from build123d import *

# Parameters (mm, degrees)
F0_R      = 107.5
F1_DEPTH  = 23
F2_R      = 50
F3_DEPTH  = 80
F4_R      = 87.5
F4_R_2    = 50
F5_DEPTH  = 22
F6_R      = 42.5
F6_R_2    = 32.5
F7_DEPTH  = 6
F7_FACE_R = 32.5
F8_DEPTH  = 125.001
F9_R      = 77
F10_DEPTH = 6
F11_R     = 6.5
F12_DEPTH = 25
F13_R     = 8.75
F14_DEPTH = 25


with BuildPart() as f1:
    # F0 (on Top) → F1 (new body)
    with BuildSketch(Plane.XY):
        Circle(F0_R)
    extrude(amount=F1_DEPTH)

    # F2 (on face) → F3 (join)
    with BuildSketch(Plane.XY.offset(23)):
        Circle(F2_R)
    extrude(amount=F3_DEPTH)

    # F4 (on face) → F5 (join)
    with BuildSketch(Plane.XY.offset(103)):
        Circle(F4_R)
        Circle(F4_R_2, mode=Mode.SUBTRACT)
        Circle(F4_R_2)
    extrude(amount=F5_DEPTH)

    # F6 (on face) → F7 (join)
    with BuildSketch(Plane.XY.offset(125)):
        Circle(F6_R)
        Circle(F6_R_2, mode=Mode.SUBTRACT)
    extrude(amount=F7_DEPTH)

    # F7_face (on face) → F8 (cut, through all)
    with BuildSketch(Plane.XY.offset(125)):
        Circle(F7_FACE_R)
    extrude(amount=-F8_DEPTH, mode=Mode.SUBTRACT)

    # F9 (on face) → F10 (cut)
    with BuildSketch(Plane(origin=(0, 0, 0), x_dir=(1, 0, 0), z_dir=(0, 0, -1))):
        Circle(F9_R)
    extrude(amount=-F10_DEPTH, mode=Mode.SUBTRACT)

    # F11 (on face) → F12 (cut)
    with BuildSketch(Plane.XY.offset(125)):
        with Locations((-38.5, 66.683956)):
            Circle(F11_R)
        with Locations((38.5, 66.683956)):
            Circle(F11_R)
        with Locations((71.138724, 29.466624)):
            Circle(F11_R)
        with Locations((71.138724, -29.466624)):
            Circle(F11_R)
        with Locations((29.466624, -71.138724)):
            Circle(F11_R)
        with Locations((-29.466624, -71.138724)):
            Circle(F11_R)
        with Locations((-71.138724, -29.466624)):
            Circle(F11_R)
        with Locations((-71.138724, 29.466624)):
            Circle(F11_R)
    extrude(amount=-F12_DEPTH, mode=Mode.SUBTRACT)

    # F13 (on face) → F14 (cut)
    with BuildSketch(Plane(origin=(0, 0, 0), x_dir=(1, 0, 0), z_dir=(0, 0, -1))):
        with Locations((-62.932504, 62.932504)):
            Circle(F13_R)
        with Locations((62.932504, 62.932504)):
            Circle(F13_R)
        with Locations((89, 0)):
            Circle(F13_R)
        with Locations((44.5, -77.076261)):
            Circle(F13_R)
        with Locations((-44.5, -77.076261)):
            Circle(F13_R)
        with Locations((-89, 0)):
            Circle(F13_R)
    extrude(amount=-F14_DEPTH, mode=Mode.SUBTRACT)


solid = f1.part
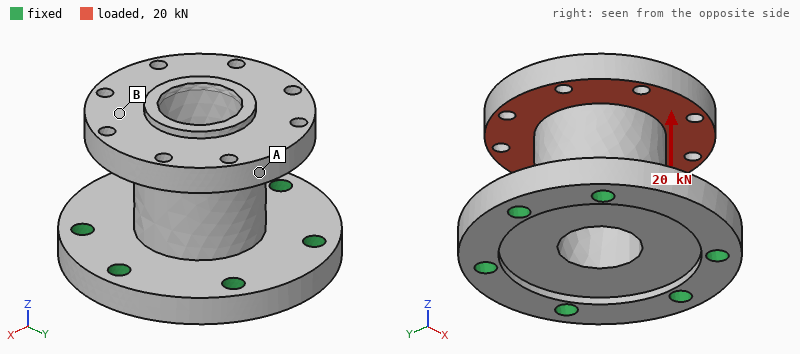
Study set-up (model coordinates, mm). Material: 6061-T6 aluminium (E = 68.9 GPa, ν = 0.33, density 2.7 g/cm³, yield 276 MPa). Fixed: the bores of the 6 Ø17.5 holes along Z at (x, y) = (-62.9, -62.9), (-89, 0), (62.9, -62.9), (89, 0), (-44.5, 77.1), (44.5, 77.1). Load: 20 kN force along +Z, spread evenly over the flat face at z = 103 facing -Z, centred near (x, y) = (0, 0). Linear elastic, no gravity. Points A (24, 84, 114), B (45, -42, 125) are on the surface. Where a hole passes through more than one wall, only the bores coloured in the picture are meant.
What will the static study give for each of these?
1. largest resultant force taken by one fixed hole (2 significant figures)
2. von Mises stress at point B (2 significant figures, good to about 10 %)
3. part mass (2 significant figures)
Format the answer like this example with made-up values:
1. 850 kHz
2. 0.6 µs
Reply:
1. 4.3 kN
2. 6.3 MPa
3. 3.9 kg
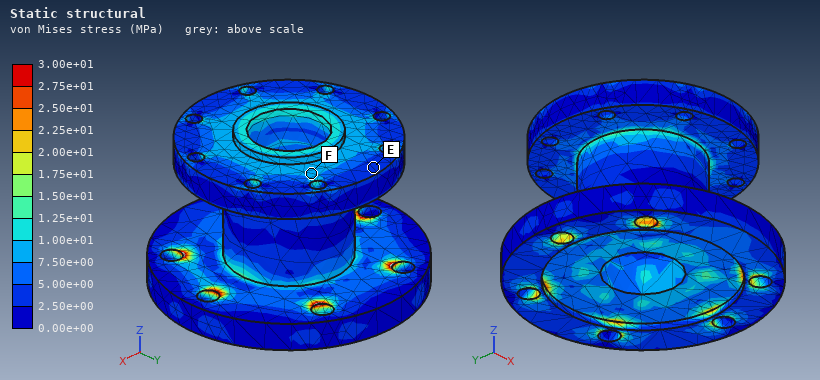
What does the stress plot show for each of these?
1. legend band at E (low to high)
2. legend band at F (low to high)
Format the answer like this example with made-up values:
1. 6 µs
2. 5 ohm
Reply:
1. 2.50e+00 to 5.00e+00 MPa
2. 7.50e+00 to 1.00e+01 MPa
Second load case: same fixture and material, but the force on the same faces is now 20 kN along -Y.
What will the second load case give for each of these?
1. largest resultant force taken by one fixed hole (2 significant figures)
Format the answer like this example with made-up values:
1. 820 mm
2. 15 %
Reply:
1. 9.2 kN
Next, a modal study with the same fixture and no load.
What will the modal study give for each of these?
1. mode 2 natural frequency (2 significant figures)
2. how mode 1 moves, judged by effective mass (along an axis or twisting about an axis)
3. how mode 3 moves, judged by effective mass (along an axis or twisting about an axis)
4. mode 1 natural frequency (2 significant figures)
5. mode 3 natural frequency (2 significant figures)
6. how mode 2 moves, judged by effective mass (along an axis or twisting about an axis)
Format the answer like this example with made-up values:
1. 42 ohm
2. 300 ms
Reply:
1. 1500 Hz
2. along Y
3. along Z
4. 1400 Hz
5. 2900 Hz
6. along X
